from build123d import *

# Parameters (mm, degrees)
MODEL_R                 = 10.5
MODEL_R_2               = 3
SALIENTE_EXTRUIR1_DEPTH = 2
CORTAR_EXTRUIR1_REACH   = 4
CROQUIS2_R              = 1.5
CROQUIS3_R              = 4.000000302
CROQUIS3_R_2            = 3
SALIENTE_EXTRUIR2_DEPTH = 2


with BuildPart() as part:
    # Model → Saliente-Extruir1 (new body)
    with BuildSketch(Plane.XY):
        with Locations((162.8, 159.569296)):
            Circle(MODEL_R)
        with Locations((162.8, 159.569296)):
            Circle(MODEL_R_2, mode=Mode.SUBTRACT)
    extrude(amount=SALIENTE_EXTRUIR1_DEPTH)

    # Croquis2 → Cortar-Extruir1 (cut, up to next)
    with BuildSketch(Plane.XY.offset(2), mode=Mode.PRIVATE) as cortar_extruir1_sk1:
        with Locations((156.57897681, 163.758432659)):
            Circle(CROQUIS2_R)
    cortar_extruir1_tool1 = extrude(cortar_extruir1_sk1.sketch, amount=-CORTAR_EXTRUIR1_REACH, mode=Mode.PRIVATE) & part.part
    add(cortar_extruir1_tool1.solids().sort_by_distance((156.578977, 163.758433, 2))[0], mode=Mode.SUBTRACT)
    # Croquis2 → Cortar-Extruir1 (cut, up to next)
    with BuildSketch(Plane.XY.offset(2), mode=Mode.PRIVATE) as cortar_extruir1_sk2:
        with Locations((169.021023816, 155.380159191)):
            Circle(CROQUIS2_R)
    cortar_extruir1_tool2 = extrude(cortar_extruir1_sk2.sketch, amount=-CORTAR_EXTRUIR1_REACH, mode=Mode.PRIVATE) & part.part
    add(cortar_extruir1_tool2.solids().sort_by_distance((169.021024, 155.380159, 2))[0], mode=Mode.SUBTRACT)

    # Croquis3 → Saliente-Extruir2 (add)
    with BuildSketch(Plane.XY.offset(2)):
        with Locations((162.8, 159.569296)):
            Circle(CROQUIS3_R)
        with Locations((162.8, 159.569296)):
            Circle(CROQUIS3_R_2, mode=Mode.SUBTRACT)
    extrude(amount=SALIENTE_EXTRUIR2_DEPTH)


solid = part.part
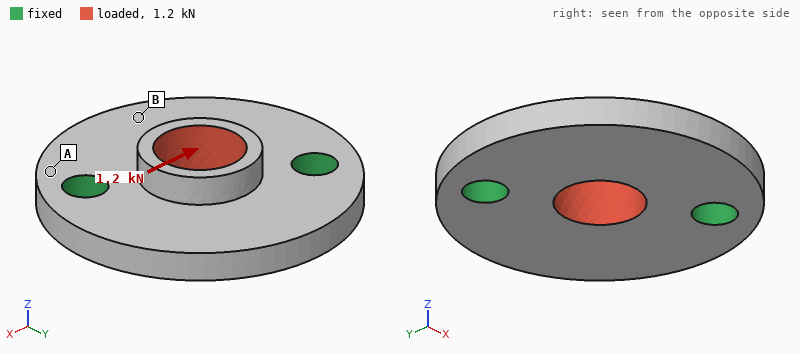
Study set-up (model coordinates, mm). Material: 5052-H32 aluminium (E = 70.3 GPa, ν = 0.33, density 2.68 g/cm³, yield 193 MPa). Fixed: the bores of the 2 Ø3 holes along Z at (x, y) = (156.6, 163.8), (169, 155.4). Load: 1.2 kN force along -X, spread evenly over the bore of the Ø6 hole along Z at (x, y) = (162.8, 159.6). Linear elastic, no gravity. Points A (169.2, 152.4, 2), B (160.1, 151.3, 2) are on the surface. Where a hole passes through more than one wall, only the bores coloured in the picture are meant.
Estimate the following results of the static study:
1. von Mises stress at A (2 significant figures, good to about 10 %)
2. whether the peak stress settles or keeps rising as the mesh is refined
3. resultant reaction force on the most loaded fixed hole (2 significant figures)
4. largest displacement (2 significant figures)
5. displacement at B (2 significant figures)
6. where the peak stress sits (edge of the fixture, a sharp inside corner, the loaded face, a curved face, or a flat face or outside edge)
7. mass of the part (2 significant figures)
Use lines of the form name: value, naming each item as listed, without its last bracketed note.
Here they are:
von Mises stress at A: 24 MPa
whether the peak stress settles or keeps rising as the mesh is refined: keeps rising
resultant reaction force on the most loaded fixed hole: 610 N
largest displacement: 12 µm
displacement at B: 9.1 µm
where the peak stress sits: edge of the fixture
mass of the part: 1.7 g
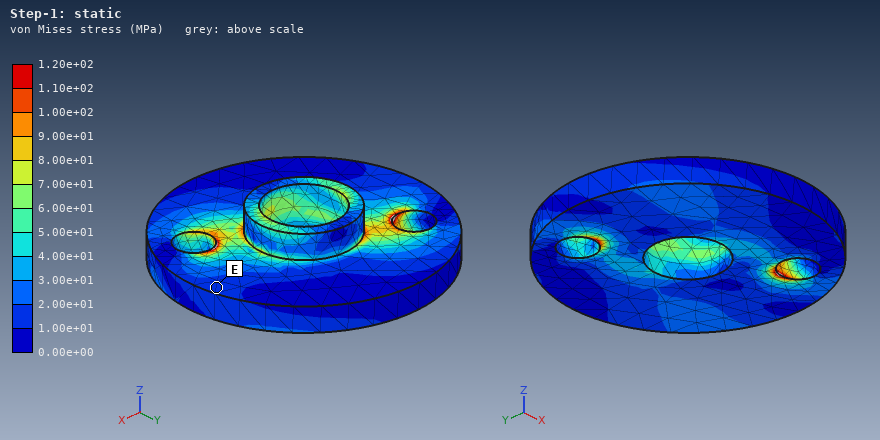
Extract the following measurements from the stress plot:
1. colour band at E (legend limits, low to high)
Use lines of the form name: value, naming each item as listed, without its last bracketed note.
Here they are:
colour band at E: 1.00e+01 to 2.00e+01 MPa
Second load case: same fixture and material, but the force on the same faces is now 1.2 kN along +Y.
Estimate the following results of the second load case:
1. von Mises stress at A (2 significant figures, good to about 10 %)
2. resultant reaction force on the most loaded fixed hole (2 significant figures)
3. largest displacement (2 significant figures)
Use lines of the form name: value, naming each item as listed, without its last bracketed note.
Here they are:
von Mises stress at A: 22 MPa
resultant reaction force on the most loaded fixed hole: 600 N
largest displacement: 18 µm
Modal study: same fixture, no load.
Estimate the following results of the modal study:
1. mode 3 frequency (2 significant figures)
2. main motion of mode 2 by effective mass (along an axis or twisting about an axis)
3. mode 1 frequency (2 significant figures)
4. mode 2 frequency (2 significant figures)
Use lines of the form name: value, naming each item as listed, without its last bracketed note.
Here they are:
mode 3 frequency: 43 kHz
main motion of mode 2 by effective mass: along Z
mode 1 frequency: 17 kHz
mode 2 frequency: 20 kHz
